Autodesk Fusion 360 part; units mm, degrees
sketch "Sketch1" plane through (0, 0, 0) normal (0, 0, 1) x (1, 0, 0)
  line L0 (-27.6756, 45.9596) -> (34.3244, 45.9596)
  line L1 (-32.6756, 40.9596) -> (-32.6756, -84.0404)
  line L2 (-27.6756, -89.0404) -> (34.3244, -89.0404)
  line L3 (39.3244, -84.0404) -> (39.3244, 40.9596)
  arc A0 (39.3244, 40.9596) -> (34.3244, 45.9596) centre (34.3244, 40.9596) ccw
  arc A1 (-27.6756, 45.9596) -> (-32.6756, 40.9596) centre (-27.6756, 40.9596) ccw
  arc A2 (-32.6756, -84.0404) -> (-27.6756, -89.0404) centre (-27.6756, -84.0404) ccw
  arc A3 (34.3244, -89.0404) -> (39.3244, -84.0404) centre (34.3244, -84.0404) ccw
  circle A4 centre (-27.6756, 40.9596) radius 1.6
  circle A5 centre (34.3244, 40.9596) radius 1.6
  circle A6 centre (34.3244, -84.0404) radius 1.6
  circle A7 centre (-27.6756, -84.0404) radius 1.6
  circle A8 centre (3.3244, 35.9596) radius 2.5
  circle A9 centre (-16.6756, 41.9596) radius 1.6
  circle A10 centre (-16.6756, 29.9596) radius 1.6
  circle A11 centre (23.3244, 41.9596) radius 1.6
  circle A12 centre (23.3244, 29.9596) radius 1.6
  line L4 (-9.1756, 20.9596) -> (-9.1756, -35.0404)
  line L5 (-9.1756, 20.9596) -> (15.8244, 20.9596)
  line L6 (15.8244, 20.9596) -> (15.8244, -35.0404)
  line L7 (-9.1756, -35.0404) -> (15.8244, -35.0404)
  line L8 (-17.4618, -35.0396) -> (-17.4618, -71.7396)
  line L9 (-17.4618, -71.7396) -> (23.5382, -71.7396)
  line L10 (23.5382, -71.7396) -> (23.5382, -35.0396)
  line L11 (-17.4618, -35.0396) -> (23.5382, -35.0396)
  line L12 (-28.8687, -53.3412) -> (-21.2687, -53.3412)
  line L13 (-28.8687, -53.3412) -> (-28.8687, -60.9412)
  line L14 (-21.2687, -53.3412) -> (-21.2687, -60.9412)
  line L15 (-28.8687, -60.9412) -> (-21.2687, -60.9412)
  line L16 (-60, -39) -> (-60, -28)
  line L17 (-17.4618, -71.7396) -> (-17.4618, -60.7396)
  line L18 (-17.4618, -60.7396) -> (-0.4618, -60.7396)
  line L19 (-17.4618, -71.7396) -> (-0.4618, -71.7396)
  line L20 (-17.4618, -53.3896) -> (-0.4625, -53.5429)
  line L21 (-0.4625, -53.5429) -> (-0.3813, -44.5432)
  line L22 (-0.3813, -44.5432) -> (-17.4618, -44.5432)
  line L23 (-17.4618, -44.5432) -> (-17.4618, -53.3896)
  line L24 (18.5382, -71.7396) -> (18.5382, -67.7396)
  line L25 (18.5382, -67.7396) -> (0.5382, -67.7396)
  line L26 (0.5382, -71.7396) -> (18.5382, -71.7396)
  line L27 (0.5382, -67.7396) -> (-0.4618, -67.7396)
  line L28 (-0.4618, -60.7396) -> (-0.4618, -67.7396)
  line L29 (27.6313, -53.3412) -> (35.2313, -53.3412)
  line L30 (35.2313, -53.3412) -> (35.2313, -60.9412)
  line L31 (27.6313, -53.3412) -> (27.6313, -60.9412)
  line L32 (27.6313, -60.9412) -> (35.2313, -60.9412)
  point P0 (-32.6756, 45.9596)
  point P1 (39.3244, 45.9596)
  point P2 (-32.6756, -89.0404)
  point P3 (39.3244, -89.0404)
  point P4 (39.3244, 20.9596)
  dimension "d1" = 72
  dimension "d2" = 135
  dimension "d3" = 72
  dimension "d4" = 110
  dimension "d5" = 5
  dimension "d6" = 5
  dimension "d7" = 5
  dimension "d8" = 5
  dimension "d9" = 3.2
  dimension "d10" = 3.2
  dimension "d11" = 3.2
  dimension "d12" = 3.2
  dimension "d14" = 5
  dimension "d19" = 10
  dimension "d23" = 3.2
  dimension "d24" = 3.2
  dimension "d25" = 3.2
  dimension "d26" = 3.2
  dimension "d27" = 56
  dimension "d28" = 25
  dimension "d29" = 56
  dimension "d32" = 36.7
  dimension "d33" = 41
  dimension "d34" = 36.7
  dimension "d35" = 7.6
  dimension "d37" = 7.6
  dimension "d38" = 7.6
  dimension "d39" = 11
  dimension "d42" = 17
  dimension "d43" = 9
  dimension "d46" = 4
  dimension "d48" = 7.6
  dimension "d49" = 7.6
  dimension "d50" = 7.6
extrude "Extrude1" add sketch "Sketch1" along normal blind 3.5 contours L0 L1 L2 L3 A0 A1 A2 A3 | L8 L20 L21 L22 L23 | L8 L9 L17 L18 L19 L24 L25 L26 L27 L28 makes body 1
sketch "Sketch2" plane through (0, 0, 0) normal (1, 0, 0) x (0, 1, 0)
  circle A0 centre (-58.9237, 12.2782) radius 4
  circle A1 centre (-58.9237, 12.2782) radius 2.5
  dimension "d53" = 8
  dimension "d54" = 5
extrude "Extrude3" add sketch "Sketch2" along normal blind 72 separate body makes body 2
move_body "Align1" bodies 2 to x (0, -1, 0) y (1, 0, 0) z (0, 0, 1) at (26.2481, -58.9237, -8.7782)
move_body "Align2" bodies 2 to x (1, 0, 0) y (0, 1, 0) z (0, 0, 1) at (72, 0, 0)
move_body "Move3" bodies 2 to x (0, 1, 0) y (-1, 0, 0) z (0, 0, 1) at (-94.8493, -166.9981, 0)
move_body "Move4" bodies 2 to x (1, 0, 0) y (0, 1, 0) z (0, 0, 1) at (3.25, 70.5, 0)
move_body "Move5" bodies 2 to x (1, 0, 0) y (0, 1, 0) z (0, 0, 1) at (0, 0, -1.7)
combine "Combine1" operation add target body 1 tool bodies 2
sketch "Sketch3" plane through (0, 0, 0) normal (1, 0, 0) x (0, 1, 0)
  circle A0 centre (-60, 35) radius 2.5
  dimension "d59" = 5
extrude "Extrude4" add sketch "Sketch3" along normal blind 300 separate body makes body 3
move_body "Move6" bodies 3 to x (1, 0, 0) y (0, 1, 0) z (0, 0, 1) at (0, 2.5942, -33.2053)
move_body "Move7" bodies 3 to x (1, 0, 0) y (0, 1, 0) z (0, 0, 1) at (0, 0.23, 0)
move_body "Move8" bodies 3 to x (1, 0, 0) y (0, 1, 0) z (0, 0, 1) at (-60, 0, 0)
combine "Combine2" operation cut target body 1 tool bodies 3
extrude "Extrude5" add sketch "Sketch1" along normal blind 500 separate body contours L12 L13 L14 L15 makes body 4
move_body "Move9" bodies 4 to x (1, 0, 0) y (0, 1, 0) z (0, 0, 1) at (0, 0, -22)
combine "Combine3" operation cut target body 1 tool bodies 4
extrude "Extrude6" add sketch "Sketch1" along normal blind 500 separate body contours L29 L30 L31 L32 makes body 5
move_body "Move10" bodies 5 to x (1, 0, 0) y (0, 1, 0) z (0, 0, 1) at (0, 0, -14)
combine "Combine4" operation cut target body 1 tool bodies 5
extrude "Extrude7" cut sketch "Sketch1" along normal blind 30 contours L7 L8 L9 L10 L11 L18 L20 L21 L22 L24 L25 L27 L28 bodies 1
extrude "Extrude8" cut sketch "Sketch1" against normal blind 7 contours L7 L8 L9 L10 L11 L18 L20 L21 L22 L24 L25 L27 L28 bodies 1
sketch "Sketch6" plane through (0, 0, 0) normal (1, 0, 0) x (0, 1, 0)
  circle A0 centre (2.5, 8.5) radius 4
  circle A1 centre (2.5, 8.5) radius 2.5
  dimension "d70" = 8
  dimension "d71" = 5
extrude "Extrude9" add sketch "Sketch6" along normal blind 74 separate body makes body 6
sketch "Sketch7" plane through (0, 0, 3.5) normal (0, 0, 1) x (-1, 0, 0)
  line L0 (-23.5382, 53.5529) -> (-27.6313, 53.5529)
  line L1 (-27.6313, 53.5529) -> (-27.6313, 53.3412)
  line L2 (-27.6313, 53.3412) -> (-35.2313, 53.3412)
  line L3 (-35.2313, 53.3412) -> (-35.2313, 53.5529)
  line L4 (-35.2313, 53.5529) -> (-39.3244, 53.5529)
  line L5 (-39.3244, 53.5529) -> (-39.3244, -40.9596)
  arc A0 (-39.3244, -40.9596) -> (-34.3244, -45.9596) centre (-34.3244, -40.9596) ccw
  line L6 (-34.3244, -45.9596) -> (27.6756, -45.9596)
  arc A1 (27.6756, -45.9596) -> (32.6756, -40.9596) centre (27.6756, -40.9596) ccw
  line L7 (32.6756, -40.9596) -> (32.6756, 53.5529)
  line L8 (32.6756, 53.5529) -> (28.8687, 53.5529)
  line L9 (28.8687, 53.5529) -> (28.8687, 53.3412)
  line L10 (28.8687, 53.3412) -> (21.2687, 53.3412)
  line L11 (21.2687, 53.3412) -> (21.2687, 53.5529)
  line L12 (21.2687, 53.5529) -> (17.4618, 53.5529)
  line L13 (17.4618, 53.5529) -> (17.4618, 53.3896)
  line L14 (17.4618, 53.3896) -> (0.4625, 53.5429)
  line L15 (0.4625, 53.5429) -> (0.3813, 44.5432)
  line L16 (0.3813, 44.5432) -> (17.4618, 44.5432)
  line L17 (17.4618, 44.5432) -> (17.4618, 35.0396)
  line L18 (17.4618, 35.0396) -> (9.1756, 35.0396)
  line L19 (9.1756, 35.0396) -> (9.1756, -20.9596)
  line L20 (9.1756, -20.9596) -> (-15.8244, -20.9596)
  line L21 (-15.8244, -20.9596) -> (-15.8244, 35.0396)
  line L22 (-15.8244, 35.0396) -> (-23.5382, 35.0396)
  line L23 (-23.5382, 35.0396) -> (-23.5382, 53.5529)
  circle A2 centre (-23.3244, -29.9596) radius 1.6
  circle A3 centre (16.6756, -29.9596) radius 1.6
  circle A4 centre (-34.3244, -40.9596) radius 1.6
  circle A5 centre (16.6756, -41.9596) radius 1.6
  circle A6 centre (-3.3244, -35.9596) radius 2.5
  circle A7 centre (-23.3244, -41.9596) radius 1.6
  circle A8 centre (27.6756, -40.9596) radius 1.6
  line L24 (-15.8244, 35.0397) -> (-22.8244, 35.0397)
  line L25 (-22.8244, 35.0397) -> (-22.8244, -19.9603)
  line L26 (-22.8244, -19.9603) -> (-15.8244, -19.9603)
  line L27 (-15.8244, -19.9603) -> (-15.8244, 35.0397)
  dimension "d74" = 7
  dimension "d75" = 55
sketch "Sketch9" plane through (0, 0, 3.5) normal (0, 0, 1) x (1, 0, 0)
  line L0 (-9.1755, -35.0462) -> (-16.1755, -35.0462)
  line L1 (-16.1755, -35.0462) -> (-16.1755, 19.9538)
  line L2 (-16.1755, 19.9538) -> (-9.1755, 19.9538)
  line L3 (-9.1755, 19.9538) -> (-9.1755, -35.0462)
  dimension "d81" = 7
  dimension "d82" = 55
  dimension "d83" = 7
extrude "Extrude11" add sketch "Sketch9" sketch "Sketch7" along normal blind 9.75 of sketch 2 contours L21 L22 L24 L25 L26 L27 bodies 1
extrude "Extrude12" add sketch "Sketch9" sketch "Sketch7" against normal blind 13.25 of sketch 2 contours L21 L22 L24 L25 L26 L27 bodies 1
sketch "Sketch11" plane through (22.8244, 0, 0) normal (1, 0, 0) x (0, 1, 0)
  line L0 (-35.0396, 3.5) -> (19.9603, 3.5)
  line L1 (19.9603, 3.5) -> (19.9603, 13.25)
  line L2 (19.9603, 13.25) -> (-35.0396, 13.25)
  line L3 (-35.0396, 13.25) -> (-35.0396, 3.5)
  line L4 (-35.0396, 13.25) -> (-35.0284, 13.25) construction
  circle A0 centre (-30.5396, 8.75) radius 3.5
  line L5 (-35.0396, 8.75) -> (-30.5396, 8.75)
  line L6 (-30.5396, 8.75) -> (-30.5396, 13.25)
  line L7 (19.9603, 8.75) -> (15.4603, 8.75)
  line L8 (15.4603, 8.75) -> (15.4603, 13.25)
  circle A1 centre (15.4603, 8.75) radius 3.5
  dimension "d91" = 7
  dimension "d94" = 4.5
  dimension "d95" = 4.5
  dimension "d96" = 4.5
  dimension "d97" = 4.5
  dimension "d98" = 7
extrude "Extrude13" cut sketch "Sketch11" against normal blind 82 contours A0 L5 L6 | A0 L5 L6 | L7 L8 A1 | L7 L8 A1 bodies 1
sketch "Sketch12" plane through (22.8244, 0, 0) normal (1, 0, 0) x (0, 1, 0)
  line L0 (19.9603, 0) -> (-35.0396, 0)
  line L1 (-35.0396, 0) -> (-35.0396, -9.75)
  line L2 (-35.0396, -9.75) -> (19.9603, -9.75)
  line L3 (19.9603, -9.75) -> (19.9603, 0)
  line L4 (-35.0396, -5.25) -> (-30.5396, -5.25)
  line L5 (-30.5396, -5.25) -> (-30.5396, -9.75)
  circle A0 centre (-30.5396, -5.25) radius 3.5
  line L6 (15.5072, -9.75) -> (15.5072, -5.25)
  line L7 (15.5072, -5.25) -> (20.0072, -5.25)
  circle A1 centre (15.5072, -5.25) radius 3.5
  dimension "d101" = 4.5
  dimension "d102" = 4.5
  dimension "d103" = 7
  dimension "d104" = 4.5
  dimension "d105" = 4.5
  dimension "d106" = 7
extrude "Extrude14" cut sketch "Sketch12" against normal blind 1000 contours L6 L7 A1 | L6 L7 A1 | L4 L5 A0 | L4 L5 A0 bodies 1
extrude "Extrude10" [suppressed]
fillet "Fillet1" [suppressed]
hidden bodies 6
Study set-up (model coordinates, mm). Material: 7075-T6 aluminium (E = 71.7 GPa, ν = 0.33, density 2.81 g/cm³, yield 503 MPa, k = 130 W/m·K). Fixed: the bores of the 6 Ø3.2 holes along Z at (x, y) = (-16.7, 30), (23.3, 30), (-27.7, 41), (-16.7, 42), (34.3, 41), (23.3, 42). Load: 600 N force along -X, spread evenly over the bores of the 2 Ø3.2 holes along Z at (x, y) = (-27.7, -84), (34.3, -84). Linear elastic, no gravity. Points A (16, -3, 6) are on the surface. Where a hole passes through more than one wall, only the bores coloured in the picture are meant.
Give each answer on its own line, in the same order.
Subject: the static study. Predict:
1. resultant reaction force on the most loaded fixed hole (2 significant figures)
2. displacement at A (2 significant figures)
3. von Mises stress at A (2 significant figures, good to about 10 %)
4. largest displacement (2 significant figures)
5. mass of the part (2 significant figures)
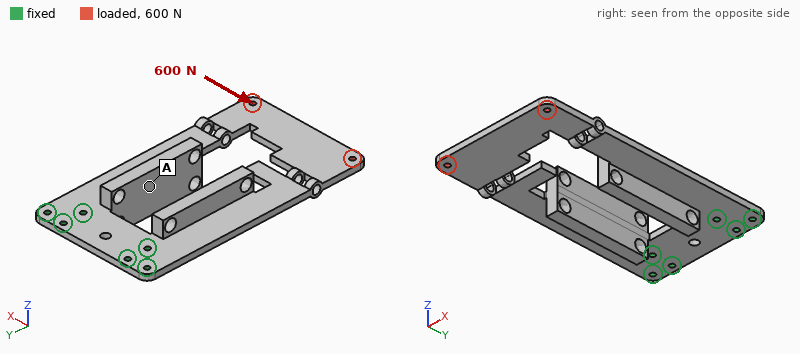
1.2 kN
0.051 mm
13 MPa
0.31 mm
110 g
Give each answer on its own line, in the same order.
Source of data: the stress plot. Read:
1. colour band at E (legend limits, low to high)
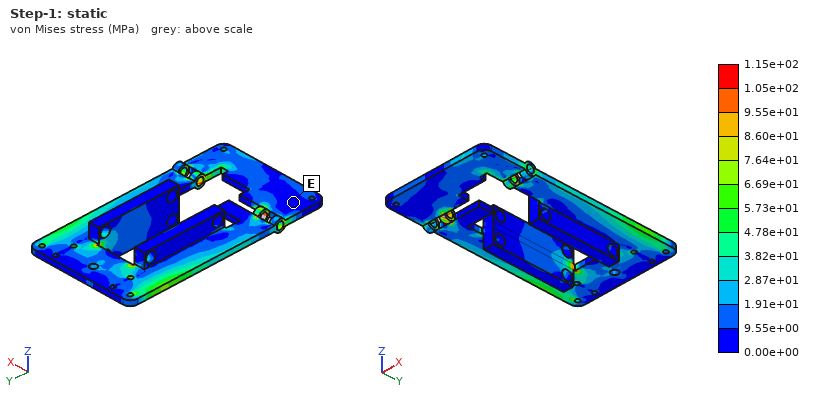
0.00e+00 to 9.55e+00 MPa
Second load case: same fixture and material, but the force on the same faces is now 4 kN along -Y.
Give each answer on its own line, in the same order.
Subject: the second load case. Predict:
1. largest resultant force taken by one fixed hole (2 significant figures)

1.2 kN
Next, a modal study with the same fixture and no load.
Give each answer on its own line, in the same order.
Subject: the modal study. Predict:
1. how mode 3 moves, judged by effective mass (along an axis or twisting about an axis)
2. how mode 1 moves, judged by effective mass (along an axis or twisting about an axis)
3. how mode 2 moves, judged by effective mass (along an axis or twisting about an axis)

along Z
along Z
twisting about Y
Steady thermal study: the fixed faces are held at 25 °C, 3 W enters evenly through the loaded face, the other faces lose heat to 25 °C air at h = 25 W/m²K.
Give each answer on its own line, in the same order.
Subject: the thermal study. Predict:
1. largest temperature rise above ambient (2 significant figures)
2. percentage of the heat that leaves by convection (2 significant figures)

12 K
61 %
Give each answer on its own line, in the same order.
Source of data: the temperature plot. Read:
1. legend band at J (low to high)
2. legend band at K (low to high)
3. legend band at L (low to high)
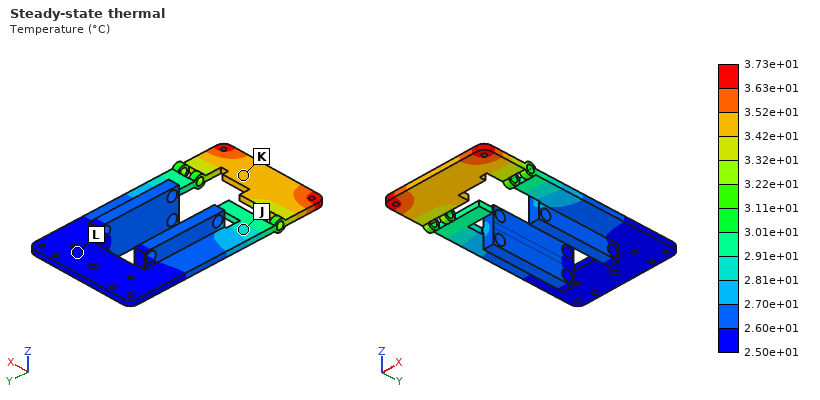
2.81e+01 to 2.91e+01 °C
3.42e+01 to 3.52e+01 °C
2.50e+01 to 2.60e+01 °C
